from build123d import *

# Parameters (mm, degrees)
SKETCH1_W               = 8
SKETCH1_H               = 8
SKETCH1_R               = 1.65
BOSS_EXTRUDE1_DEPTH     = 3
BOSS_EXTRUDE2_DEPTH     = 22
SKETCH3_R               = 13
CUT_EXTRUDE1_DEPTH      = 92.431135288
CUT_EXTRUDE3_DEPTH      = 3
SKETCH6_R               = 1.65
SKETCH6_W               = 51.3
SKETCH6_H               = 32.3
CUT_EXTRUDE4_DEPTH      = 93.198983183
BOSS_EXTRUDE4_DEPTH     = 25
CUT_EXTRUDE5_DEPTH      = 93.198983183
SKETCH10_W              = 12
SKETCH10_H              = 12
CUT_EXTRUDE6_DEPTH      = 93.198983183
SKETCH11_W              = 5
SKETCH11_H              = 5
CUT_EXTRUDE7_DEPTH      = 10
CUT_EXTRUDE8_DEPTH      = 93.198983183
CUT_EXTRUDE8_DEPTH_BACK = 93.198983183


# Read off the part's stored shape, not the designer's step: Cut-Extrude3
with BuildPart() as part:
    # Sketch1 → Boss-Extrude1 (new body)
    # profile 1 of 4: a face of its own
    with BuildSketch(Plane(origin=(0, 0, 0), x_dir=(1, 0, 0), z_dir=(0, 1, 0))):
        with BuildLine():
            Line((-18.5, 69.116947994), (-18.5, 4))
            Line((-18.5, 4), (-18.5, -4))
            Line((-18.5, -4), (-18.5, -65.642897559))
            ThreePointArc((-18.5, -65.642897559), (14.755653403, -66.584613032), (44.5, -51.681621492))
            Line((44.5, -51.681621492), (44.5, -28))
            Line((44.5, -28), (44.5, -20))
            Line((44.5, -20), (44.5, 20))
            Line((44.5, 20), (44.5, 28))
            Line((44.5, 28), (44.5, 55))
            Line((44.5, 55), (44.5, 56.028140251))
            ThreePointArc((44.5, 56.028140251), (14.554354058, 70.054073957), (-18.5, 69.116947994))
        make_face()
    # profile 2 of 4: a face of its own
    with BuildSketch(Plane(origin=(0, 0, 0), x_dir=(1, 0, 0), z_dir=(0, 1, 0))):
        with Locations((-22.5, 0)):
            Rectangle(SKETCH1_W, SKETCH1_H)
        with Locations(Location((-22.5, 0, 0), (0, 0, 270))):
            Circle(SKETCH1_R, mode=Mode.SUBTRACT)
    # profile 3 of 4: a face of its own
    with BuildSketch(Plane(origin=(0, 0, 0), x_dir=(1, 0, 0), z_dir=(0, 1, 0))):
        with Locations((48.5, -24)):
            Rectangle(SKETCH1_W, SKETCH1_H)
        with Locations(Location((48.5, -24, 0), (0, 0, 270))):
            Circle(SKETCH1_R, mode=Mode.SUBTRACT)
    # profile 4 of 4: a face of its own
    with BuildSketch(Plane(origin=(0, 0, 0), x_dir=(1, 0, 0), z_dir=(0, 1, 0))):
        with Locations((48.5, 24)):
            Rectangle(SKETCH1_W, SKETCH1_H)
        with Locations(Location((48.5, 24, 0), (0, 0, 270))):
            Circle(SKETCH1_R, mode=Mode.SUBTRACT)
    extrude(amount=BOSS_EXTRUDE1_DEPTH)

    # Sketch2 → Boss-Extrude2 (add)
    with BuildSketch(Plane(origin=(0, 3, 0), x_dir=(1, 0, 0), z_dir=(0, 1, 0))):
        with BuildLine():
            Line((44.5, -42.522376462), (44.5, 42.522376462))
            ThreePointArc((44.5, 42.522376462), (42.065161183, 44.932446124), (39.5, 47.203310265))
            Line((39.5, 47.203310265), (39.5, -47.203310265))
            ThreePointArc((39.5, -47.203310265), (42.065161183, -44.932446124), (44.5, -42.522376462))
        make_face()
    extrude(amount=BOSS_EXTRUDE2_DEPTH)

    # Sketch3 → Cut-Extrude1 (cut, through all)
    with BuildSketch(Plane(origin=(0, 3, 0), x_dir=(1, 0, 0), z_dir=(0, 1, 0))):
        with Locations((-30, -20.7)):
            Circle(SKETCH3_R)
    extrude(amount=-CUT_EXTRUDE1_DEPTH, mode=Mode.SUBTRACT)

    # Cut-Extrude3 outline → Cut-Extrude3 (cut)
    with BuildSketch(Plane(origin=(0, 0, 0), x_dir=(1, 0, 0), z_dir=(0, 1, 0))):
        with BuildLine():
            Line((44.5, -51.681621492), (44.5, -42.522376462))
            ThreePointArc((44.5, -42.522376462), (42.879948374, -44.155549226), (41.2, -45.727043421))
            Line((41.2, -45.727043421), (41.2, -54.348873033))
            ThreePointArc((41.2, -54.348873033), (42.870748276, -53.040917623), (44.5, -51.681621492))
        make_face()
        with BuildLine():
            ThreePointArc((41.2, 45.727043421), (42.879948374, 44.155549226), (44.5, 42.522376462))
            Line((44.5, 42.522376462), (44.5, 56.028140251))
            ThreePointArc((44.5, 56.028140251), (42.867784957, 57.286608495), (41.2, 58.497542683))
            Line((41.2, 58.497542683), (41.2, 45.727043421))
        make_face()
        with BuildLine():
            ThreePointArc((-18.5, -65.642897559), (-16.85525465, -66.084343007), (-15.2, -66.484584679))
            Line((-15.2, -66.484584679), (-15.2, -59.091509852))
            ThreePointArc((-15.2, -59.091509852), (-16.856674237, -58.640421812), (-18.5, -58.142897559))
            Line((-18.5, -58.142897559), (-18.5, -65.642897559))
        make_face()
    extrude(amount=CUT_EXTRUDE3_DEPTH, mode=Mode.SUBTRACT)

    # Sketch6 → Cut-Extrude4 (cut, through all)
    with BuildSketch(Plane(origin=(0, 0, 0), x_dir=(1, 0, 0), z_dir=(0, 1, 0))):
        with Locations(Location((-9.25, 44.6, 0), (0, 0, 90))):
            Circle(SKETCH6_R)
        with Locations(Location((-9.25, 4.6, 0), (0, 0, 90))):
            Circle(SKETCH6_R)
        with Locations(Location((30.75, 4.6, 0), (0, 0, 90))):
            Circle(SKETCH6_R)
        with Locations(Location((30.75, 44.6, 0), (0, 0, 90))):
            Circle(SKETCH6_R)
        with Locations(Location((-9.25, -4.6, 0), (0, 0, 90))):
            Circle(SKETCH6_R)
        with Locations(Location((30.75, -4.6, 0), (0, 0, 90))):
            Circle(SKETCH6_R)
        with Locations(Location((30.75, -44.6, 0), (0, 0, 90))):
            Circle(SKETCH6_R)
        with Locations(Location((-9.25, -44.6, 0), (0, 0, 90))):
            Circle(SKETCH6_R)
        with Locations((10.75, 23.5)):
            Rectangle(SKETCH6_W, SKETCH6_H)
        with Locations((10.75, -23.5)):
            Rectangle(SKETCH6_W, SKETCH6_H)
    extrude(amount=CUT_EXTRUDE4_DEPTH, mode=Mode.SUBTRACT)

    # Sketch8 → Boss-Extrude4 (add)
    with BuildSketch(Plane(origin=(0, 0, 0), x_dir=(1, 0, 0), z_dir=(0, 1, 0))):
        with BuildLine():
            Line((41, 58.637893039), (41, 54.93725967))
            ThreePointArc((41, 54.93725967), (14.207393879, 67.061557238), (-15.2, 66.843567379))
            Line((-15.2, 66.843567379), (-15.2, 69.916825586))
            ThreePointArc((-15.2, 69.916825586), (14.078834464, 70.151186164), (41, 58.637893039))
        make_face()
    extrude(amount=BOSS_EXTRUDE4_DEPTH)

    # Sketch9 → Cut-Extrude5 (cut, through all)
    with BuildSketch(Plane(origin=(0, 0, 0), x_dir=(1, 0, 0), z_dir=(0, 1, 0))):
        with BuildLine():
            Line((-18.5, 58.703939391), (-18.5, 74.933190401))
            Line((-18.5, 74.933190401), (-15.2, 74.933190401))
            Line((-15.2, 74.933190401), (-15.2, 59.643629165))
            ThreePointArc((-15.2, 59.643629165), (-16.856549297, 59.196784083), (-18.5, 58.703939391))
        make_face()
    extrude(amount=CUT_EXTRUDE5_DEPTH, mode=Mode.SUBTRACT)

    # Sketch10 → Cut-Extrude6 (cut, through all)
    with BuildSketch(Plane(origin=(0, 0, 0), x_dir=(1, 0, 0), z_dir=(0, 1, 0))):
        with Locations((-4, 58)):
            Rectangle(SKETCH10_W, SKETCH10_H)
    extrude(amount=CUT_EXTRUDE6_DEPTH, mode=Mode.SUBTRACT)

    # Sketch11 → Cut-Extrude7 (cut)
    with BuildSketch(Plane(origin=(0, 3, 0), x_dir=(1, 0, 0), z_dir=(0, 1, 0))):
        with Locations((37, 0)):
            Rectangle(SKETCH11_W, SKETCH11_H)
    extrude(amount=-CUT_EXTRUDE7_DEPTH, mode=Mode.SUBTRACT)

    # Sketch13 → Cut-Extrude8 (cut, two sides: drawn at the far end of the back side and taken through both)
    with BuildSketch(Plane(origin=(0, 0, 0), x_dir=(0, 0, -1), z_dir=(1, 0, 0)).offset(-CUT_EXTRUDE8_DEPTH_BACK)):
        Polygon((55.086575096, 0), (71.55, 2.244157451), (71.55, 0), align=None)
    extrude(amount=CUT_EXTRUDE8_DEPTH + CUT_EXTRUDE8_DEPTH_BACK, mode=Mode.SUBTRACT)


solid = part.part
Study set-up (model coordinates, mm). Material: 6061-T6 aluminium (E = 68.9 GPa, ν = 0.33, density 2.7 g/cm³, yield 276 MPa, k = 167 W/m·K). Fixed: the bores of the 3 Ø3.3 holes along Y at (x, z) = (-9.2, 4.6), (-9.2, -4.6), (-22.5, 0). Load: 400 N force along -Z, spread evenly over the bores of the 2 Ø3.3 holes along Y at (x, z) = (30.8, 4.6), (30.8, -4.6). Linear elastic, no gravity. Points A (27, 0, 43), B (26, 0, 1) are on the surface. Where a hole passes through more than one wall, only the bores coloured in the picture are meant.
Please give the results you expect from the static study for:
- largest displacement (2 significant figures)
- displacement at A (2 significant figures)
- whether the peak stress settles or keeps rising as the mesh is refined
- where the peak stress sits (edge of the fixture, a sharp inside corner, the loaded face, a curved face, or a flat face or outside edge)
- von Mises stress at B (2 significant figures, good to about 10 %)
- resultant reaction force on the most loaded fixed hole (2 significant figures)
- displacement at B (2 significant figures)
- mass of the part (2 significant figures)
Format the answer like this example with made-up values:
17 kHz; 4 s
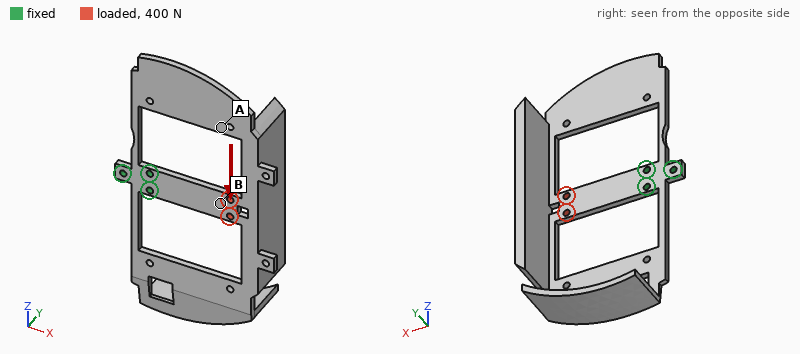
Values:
0.29 mm; 0.21 mm; keeps rising; edge of the fixture; 21 MPa; 1.5 kN; 0.12 mm; 74 g
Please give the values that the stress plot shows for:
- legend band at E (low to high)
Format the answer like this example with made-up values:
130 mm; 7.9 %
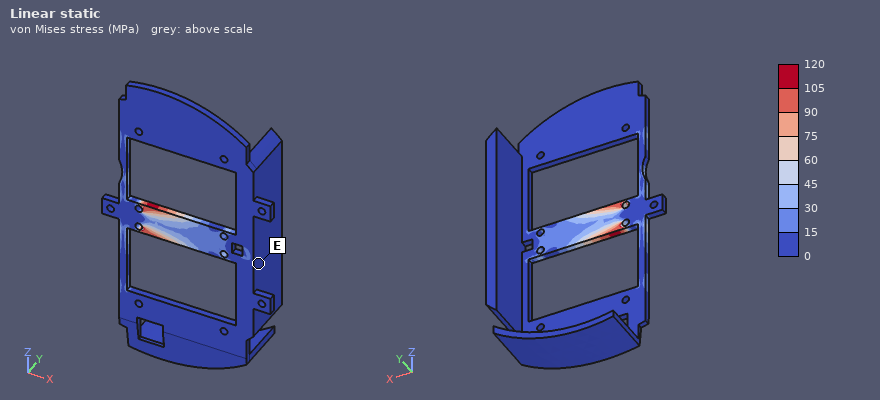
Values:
0 to 15 MPa
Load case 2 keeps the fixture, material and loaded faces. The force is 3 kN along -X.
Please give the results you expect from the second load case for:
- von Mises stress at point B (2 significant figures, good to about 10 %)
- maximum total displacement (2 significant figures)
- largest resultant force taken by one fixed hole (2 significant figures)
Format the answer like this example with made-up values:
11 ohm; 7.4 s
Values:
64 MPa; 44 µm; 1.5 kN
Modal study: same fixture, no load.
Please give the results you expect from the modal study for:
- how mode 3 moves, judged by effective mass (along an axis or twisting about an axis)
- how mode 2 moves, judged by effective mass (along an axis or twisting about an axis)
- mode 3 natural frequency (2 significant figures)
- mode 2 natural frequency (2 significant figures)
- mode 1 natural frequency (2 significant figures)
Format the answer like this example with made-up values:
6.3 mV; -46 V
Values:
along Y; along Y; 450 Hz; 210 Hz; 160 Hz
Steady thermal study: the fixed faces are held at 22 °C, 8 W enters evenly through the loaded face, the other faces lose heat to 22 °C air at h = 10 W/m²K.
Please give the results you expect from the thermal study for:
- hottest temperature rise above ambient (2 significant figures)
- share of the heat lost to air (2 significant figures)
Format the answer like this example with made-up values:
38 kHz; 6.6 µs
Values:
25 K; 32 %
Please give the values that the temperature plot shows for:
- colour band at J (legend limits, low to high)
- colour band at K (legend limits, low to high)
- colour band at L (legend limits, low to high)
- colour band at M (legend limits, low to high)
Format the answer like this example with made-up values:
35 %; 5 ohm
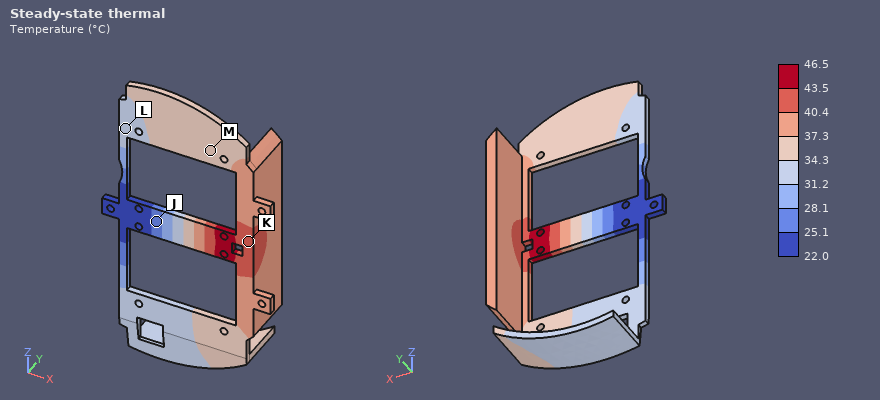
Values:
25.1 to 28.1 °C; 40.4 to 43.5 °C; 31.2 to 34.3 °C; 34.3 to 37.3 °C
